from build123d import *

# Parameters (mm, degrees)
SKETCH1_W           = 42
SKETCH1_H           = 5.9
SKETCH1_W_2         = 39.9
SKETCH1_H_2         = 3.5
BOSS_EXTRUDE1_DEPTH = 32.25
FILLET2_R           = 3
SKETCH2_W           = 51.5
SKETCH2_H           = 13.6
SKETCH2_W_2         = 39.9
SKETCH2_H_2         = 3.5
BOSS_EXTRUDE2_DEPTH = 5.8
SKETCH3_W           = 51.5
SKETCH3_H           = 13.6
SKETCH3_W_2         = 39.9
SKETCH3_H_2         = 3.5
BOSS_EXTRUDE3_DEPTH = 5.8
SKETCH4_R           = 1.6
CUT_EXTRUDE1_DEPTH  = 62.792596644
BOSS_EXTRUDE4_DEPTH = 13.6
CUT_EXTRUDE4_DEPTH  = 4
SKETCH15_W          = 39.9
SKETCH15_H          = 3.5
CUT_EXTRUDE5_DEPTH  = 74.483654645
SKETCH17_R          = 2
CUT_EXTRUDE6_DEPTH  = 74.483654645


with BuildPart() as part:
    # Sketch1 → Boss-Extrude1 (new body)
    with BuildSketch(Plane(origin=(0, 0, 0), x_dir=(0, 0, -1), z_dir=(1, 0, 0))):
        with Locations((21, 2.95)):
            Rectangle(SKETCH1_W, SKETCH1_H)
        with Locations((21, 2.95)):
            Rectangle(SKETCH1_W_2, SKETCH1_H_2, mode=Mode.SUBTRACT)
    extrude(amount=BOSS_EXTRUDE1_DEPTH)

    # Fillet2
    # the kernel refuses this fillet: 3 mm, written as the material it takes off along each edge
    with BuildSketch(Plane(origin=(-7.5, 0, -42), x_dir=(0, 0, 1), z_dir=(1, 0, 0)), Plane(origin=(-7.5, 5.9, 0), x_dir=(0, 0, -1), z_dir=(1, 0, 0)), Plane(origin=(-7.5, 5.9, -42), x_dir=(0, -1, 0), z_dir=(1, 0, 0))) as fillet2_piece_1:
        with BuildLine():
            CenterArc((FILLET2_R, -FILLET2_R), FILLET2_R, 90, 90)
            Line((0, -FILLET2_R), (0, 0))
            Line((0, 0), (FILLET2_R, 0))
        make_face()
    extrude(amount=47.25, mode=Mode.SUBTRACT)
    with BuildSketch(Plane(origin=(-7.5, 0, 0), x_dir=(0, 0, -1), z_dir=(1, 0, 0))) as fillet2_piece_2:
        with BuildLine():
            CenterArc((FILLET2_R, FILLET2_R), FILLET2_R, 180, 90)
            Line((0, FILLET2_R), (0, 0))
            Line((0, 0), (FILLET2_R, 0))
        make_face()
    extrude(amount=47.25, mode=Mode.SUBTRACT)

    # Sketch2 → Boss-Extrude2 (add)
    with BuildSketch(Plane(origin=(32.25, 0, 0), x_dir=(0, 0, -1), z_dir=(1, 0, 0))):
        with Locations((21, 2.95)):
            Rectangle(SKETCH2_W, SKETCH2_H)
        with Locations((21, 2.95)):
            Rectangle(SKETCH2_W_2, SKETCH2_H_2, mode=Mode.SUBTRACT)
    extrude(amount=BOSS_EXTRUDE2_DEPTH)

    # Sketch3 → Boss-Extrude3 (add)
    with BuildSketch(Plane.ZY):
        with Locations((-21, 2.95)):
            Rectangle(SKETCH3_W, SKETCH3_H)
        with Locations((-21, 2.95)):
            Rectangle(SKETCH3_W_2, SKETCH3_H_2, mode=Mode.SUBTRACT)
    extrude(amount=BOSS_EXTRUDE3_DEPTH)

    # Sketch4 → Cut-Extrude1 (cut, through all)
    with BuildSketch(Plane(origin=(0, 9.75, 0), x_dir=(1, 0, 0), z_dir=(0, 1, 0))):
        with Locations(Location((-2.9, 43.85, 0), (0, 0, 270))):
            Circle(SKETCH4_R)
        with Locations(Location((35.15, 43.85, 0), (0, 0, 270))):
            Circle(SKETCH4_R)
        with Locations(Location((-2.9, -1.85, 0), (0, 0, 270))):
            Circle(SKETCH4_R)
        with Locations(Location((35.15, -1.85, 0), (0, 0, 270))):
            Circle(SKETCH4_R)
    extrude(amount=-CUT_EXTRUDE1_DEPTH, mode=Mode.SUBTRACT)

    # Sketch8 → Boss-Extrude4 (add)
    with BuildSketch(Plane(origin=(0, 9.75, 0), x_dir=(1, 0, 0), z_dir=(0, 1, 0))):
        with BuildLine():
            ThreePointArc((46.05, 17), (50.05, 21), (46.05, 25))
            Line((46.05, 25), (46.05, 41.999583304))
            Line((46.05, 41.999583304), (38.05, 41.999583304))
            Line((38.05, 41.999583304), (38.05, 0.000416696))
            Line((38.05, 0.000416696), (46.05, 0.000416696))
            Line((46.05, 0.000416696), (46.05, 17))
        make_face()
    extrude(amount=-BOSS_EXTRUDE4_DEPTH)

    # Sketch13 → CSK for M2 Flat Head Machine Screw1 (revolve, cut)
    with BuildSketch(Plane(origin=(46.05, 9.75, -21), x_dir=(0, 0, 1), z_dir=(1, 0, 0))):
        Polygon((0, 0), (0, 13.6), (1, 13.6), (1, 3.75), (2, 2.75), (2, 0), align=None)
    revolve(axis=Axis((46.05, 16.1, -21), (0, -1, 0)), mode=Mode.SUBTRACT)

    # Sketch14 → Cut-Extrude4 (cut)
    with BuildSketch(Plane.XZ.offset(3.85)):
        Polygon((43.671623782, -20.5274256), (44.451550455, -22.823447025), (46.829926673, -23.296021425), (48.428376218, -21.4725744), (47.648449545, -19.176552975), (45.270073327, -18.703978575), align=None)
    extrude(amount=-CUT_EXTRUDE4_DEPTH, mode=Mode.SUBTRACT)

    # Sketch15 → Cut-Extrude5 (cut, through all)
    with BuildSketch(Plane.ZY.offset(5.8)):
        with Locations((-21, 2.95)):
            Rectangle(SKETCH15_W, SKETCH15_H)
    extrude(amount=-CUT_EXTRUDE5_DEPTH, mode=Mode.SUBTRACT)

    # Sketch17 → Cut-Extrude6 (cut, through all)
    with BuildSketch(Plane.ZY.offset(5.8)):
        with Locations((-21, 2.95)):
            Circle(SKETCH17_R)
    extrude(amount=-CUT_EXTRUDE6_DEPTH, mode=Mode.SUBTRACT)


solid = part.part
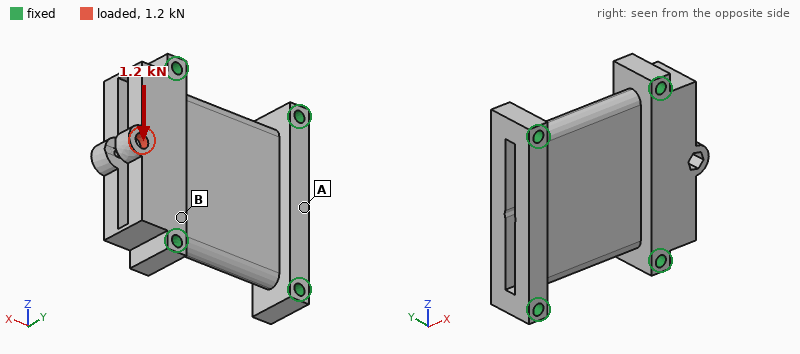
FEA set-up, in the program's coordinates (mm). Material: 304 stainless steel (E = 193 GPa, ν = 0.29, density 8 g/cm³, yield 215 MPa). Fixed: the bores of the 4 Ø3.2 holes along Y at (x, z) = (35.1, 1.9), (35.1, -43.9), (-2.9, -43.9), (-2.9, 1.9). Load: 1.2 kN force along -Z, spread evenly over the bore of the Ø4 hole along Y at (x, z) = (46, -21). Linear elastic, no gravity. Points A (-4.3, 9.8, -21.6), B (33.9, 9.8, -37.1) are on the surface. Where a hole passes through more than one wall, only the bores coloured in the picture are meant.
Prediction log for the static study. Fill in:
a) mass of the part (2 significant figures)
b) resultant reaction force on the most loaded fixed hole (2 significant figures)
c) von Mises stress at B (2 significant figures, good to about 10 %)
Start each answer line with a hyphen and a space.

- 100 g
- 660 N
- 9.2 MPa
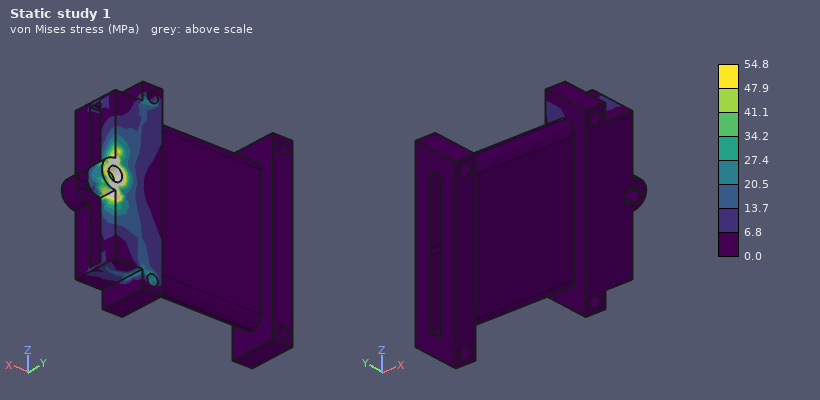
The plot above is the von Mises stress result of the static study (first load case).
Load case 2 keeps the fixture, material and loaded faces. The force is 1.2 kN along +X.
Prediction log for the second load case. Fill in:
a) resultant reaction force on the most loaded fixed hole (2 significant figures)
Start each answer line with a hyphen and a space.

- 550 N
